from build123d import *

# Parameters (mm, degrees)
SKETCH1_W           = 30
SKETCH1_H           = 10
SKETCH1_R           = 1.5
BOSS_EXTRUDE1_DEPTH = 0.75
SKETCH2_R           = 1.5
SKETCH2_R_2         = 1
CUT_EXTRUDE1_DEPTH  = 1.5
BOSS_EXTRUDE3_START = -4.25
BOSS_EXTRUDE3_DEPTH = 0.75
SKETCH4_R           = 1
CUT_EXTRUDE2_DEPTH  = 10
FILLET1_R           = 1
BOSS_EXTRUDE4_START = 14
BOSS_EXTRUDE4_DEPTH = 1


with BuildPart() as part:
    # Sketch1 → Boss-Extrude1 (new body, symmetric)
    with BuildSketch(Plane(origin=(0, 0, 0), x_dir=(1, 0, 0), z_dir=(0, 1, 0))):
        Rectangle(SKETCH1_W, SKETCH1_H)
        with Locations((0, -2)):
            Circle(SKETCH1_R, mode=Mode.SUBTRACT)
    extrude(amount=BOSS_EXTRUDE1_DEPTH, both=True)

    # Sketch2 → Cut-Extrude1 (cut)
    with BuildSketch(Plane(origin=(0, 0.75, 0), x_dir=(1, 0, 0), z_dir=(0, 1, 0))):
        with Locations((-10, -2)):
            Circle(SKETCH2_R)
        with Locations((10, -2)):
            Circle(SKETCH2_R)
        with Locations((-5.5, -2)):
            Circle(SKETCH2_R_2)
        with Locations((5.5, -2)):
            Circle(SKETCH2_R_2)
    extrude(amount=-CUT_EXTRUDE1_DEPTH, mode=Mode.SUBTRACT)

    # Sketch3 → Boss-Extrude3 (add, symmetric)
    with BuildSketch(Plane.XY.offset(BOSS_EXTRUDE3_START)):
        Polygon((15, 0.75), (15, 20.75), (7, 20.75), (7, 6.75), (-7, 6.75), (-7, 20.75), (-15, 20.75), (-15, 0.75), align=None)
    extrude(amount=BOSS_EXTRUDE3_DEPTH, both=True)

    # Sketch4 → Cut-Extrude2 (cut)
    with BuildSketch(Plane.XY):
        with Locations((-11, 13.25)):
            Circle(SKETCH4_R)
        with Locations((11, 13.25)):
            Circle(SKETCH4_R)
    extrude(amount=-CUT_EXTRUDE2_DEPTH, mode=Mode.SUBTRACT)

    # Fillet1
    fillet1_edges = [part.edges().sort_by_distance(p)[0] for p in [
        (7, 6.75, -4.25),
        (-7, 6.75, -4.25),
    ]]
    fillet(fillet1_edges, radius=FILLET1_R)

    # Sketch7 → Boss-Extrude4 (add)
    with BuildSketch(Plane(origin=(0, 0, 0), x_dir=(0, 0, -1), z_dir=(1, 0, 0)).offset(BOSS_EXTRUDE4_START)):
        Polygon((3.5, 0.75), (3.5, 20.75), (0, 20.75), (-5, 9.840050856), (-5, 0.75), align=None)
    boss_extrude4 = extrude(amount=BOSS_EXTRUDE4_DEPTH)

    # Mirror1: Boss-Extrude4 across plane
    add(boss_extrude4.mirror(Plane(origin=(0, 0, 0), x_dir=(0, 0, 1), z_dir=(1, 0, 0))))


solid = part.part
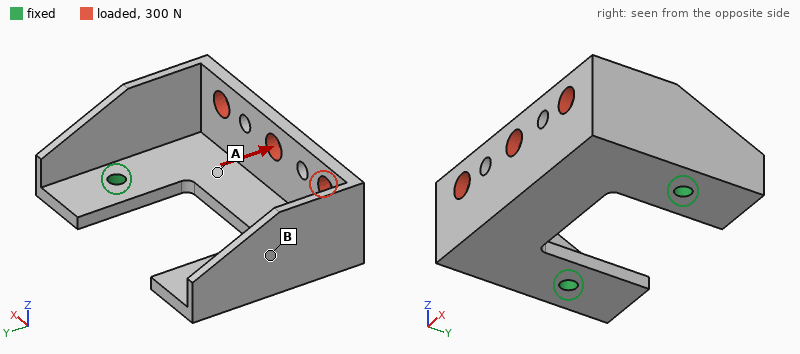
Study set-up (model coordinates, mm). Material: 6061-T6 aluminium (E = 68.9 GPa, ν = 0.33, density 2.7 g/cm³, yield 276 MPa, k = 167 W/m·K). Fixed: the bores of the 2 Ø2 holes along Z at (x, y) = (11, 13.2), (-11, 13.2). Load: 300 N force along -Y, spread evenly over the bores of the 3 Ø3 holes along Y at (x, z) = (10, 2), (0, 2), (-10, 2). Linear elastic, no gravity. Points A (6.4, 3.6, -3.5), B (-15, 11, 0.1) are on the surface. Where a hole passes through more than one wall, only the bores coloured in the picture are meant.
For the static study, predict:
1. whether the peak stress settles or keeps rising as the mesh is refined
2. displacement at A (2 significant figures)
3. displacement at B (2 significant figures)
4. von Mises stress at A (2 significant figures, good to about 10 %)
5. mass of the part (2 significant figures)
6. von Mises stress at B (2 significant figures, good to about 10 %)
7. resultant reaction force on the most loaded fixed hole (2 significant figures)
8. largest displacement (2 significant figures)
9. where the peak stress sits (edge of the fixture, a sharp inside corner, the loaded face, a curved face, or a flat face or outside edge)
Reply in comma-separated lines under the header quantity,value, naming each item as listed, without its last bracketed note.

quantity,value
whether the peak stress settles or keeps rising as the mesh is refined,keeps rising
displacement at A,0.063 mm
displacement at B,0.040 mm
von Mises stress at A,68 MPa
mass of the part,3.5 g
von Mises stress at B,35 MPa
resultant reaction force on the most loaded fixed hole,150 N
largest displacement,0.24 mm
where the peak stress sits,edge of the fixture
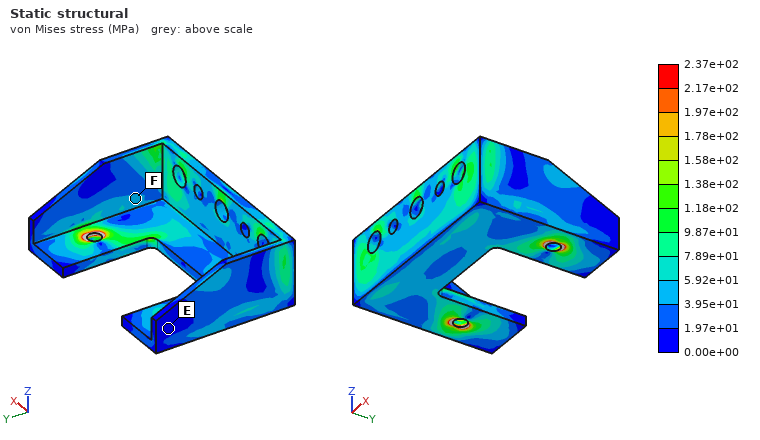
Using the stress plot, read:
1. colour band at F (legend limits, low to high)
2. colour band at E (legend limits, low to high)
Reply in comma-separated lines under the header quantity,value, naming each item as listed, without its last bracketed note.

quantity,value
colour band at F,3.95e+01 to 5.92e+01 MPa
colour band at E,0.00e+00 to 1.97e+01 MPa
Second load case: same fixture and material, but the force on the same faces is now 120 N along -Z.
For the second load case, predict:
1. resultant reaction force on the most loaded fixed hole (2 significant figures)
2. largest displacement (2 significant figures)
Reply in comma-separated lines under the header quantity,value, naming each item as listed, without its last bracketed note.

quantity,value
resultant reaction force on the most loaded fixed hole,60 N
largest displacement,0.12 mm
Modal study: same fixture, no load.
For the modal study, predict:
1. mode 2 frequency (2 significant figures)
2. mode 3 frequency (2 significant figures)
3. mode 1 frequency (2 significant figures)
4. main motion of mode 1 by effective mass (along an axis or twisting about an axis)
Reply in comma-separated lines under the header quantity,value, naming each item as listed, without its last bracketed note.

quantity,value
mode 2 frequency,5900 Hz
mode 3 frequency,13 kHz
mode 1 frequency,4200 Hz
main motion of mode 1 by effective mass,along Z
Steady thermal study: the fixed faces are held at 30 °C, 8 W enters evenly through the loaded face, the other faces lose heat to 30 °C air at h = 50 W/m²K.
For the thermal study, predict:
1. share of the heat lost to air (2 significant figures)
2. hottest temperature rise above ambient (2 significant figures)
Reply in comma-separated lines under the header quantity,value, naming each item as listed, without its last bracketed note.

quantity,value
share of the heat lost to air,14 %
hottest temperature rise above ambient,23 K
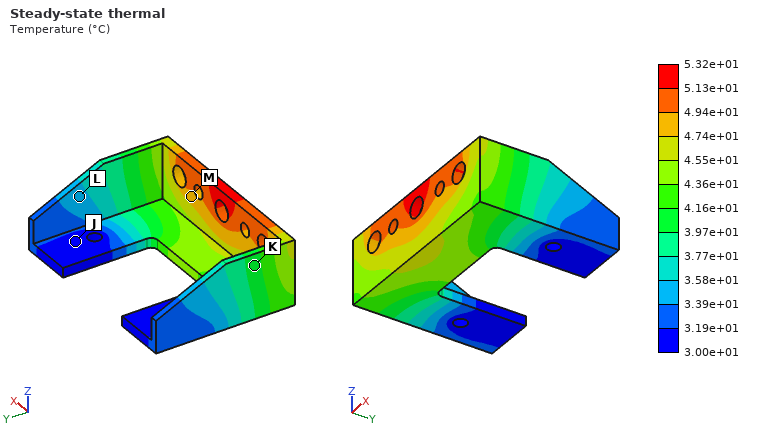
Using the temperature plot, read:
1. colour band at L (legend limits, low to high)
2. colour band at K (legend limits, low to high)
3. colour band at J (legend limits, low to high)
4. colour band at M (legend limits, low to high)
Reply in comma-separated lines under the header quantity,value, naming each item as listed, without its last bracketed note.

quantity,value
colour band at L,3.39e+01 to 3.58e+01 °C
colour band at K,3.97e+01 to 4.16e+01 °C
colour band at J,3.00e+01 to 3.19e+01 °C
colour band at M,4.74e+01 to 4.94e+01 °C
